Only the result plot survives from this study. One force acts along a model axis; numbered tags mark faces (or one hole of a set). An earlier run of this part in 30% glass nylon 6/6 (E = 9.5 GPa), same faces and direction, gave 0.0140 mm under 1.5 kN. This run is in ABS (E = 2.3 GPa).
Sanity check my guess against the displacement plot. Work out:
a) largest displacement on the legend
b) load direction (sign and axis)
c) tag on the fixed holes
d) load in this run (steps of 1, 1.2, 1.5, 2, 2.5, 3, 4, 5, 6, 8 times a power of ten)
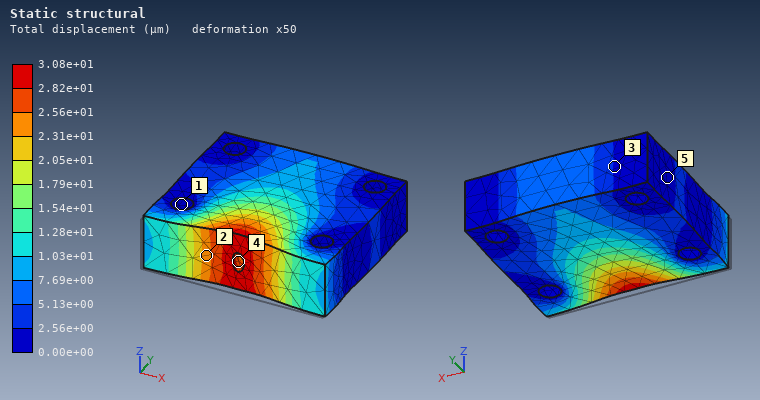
3.08e+01 µm
+Y
1
800 N
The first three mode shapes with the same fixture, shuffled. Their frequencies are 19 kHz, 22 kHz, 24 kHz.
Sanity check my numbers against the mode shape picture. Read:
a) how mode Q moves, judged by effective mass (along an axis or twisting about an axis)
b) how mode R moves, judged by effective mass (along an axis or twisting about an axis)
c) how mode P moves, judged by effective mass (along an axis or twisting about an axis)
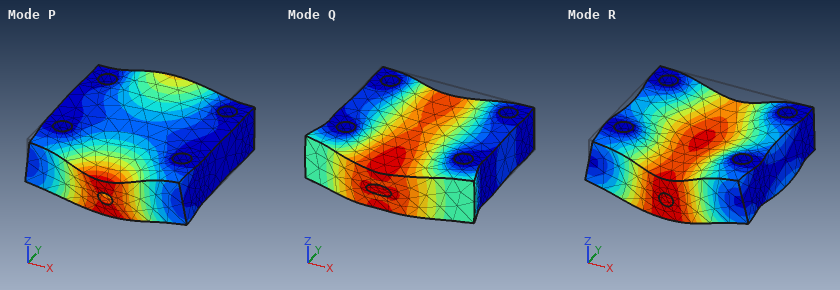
along Y
along Z
twisting about X
